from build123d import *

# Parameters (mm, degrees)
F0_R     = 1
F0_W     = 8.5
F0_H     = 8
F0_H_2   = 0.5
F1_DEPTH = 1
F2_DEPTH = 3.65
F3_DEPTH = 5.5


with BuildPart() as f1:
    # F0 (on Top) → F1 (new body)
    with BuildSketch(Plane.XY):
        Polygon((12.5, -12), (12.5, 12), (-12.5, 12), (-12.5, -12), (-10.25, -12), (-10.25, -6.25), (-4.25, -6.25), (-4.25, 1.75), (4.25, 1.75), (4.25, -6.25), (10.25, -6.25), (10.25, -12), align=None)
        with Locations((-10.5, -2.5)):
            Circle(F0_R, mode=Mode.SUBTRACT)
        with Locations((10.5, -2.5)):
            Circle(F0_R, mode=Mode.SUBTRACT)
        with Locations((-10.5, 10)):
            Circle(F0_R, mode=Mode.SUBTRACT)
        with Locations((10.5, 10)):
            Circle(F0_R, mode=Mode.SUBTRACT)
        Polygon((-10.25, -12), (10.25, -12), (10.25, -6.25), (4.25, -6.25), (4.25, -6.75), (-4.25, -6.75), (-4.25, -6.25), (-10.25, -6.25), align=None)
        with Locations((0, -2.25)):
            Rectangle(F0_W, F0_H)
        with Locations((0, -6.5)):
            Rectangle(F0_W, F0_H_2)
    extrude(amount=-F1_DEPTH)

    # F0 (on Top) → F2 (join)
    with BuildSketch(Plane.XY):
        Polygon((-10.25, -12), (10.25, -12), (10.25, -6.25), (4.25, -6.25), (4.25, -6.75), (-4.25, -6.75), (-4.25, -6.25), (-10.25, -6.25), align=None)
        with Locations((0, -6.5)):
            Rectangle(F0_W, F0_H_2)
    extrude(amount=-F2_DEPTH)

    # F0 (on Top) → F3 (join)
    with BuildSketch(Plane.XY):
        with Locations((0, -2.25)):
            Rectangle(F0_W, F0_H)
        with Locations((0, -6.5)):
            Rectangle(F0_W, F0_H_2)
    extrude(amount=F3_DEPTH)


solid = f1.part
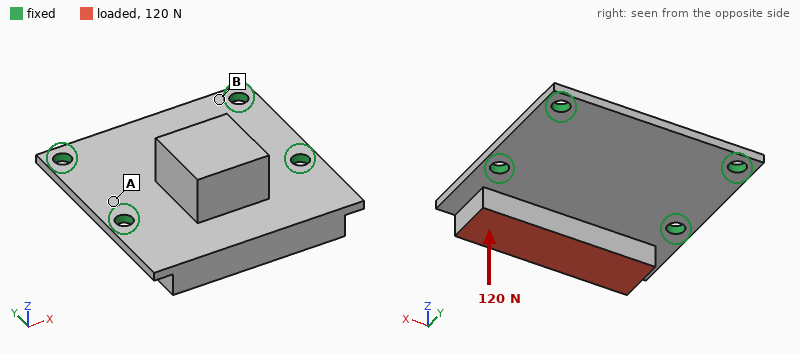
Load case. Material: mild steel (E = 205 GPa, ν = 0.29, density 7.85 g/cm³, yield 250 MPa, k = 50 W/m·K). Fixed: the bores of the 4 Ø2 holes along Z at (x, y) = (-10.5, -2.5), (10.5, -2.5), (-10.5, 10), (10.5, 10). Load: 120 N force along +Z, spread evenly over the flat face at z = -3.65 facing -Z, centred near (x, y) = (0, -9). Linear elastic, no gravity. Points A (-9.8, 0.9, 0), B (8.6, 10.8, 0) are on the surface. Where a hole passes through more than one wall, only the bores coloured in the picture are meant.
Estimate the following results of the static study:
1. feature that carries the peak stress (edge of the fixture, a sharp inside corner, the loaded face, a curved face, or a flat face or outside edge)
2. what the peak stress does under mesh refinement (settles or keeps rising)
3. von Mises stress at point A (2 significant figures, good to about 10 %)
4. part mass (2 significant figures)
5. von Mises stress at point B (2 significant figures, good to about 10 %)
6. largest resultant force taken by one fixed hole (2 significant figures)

edge of the fixture
keeps rising
14 MPa
10 g
29 MPa
75 N
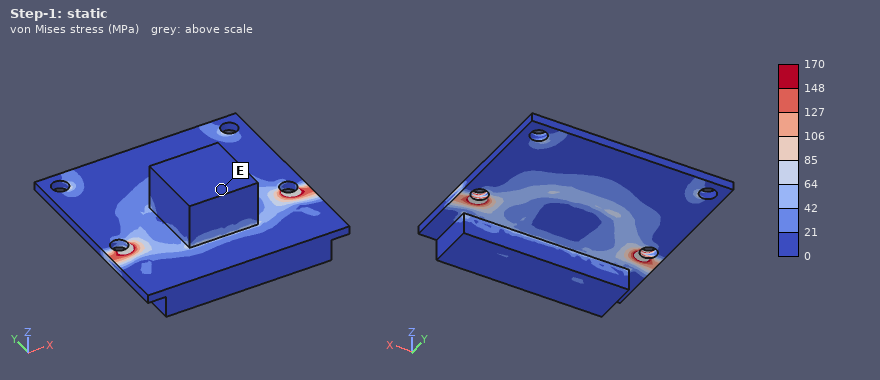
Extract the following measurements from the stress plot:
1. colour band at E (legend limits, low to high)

0 to 21 MPa
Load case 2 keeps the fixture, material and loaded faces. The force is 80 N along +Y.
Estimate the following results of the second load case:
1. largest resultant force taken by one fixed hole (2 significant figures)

32 N
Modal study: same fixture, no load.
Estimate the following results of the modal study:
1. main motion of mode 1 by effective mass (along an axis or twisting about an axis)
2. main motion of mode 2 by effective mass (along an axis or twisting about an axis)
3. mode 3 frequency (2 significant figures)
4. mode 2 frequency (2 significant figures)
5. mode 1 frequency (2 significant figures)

along Z
along Z
17 kHz
11 kHz
5700 Hz
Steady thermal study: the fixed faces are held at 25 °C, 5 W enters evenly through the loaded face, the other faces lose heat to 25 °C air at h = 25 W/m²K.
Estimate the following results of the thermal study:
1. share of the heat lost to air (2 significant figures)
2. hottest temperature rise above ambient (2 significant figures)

9.3 %
28 K
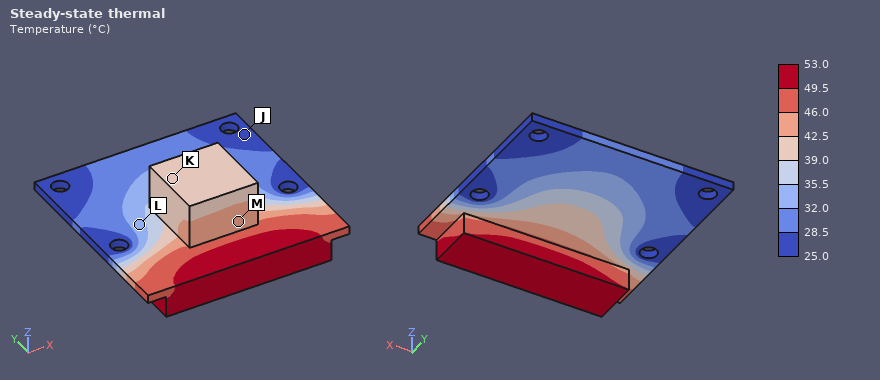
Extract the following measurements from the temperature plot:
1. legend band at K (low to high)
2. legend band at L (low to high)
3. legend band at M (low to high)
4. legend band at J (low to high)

39.0 to 42.5 °C
32.0 to 35.5 °C
42.5 to 46.0 °C
25.0 to 28.5 °C
